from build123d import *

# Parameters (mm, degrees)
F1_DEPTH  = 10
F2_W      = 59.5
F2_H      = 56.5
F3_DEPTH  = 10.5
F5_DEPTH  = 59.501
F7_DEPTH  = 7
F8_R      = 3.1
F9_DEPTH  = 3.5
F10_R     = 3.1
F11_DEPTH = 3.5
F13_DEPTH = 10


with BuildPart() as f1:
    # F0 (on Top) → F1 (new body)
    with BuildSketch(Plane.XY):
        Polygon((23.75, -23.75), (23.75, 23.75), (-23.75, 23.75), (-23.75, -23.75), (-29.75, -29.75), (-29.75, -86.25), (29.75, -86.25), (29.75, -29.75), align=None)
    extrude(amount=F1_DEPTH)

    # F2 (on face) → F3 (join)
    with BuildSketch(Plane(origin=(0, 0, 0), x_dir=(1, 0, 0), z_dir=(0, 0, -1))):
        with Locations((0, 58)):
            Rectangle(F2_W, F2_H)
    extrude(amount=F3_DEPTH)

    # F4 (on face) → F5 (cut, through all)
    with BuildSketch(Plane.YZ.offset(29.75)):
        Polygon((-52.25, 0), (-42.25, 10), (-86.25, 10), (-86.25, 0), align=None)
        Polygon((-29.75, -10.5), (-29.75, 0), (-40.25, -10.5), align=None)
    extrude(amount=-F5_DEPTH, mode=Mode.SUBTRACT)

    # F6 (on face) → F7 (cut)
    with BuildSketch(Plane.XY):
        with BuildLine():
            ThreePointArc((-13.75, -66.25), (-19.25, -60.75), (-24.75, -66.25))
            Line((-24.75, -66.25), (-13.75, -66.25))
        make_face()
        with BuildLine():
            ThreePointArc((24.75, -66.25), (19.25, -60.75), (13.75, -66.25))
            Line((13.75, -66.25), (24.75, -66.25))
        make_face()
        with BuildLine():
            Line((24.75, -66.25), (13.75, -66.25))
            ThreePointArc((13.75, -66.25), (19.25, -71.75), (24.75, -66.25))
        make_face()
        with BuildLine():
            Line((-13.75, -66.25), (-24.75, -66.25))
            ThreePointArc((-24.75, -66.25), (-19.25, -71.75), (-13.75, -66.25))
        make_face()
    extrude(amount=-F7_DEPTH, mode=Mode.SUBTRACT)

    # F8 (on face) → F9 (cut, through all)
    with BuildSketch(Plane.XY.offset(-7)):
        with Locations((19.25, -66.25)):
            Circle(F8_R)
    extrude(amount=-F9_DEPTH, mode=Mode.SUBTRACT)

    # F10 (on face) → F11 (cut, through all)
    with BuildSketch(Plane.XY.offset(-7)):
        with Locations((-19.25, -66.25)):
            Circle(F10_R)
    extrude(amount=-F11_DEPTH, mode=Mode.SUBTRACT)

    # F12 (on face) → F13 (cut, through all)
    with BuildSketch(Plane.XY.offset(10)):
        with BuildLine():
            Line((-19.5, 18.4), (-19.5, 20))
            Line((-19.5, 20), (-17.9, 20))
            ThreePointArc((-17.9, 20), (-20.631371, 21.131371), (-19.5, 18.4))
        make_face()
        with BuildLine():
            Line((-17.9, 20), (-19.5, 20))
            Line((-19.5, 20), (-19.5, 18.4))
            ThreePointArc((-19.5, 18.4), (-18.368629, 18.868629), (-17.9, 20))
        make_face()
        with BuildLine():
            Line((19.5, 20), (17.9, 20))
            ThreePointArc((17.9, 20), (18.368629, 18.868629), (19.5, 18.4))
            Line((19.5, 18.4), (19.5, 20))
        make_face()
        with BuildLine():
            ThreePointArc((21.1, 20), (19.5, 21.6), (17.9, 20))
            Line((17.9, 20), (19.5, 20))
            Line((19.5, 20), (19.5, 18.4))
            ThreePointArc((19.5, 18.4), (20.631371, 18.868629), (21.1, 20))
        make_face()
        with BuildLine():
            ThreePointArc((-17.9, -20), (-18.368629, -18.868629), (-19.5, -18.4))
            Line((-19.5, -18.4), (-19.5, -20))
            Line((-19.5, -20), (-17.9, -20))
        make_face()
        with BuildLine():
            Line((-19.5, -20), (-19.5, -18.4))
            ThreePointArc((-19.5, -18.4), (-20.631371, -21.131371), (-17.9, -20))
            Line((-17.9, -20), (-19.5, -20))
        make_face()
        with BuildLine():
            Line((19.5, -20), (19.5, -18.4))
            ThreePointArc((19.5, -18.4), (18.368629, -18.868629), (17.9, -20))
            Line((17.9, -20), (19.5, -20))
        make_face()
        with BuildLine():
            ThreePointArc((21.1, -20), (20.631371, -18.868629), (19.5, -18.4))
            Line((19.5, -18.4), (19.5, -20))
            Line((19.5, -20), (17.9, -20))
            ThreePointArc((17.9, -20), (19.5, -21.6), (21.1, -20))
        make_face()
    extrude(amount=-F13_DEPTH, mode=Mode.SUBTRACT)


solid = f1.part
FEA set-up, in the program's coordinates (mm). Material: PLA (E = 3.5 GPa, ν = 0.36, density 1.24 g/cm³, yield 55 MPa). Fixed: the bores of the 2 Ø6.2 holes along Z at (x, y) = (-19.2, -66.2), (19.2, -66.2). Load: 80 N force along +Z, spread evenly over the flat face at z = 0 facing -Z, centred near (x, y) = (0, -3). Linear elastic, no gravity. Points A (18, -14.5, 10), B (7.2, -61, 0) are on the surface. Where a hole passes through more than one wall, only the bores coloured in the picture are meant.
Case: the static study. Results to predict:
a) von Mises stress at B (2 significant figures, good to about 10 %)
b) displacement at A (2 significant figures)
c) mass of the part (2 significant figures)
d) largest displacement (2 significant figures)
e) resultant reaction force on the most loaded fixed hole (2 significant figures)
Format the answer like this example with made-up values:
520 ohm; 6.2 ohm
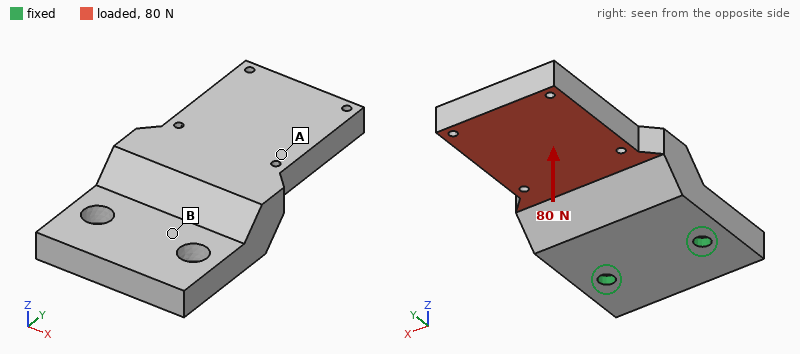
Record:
4.5 MPa; 0.70 mm; 82 g; 1.3 mm; 49 N
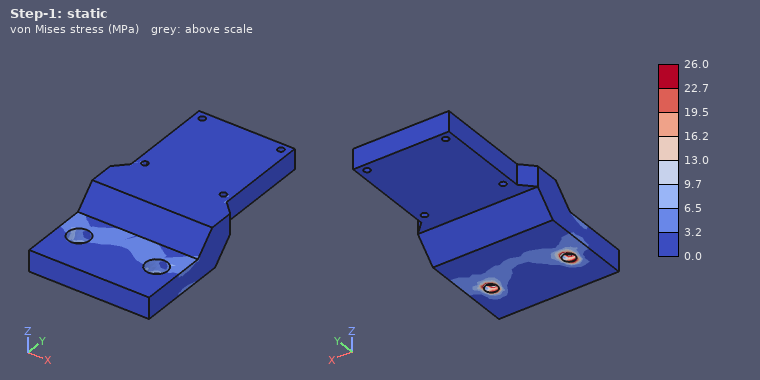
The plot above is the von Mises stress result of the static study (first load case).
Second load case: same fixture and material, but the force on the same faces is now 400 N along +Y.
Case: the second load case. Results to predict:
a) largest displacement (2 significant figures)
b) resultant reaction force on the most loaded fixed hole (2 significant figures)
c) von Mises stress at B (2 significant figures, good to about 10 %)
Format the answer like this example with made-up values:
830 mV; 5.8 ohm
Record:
0.60 mm; 200 N; 3.0 MPa
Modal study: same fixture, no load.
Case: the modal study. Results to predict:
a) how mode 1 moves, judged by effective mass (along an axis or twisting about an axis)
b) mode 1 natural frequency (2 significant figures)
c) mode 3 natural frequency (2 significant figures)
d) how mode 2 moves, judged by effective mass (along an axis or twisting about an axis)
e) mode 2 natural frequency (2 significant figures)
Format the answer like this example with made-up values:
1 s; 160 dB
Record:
along Z; 250 Hz; 1500 Hz; along X; 1200 Hz
